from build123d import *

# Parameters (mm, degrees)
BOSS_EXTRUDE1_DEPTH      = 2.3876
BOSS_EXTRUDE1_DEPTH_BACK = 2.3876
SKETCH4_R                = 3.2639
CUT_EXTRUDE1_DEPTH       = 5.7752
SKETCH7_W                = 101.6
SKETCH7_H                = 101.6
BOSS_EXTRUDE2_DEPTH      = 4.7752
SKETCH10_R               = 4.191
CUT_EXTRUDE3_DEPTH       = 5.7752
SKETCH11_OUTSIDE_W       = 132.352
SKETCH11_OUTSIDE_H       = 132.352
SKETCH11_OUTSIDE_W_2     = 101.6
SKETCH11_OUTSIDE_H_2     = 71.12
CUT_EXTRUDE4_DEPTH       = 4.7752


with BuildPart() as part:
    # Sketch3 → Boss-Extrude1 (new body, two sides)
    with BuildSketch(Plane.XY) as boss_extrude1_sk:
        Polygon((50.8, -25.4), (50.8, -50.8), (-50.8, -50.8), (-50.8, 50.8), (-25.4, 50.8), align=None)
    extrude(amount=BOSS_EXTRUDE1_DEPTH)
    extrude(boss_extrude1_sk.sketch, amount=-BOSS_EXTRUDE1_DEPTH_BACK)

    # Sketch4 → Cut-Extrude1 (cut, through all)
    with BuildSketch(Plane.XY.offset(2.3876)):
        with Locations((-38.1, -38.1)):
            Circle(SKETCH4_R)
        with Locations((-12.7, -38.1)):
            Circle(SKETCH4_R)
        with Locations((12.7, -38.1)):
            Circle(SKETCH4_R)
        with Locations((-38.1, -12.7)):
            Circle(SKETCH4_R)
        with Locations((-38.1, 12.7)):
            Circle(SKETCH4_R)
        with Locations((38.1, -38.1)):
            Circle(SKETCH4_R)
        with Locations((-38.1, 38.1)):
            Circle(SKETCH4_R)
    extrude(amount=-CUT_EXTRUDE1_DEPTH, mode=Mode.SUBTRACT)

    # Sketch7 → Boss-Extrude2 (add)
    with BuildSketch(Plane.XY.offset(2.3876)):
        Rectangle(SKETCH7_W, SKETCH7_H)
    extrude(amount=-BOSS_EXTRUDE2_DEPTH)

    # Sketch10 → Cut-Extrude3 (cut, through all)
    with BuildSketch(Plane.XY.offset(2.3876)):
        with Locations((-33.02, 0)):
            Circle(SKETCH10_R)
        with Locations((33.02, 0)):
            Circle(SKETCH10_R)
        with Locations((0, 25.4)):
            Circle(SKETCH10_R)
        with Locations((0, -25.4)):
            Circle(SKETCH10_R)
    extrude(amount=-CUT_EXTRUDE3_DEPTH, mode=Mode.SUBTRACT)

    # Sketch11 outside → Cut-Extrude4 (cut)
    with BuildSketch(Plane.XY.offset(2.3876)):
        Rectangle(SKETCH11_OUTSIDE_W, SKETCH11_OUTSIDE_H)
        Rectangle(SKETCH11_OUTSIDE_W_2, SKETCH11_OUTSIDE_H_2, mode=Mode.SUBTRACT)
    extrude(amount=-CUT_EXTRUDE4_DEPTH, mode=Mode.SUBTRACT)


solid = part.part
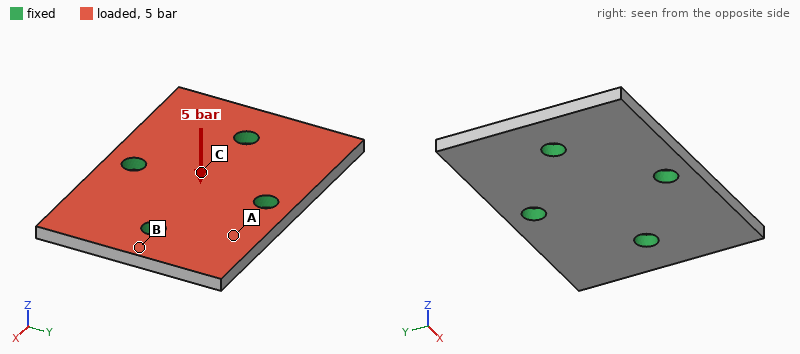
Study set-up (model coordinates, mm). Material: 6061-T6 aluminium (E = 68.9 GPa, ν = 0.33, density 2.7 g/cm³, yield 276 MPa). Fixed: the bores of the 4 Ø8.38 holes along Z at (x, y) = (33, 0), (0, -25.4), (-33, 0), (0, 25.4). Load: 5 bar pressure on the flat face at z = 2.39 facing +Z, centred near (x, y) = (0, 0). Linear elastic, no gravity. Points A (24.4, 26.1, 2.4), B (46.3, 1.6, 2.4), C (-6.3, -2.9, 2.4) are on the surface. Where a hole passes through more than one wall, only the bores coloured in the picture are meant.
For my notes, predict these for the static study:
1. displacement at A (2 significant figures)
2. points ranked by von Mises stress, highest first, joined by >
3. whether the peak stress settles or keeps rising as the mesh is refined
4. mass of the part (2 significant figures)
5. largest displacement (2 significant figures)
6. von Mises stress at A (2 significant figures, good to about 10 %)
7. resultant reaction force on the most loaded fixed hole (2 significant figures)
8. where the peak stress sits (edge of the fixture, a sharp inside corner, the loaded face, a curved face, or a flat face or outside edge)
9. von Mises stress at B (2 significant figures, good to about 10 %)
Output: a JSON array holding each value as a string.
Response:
["26 µm", "B > A > C", "keeps rising", "90 g", "85 µm", "17 MPa", "1.0 kN", "edge of the fixture", "32 MPa"]
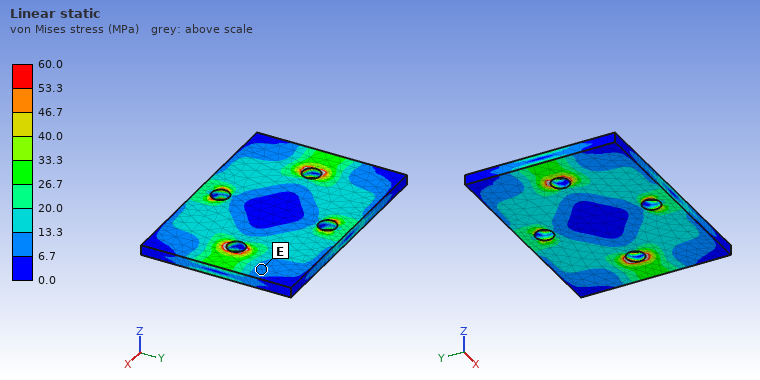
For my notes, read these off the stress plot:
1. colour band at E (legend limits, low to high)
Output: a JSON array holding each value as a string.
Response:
["6.7 to 13.3 MPa"]
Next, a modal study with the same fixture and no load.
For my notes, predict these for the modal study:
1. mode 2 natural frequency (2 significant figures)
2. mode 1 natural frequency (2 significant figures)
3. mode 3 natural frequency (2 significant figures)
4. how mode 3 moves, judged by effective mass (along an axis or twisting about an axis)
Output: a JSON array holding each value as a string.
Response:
["4500 Hz", "4500 Hz", "4800 Hz", "along Z"]
